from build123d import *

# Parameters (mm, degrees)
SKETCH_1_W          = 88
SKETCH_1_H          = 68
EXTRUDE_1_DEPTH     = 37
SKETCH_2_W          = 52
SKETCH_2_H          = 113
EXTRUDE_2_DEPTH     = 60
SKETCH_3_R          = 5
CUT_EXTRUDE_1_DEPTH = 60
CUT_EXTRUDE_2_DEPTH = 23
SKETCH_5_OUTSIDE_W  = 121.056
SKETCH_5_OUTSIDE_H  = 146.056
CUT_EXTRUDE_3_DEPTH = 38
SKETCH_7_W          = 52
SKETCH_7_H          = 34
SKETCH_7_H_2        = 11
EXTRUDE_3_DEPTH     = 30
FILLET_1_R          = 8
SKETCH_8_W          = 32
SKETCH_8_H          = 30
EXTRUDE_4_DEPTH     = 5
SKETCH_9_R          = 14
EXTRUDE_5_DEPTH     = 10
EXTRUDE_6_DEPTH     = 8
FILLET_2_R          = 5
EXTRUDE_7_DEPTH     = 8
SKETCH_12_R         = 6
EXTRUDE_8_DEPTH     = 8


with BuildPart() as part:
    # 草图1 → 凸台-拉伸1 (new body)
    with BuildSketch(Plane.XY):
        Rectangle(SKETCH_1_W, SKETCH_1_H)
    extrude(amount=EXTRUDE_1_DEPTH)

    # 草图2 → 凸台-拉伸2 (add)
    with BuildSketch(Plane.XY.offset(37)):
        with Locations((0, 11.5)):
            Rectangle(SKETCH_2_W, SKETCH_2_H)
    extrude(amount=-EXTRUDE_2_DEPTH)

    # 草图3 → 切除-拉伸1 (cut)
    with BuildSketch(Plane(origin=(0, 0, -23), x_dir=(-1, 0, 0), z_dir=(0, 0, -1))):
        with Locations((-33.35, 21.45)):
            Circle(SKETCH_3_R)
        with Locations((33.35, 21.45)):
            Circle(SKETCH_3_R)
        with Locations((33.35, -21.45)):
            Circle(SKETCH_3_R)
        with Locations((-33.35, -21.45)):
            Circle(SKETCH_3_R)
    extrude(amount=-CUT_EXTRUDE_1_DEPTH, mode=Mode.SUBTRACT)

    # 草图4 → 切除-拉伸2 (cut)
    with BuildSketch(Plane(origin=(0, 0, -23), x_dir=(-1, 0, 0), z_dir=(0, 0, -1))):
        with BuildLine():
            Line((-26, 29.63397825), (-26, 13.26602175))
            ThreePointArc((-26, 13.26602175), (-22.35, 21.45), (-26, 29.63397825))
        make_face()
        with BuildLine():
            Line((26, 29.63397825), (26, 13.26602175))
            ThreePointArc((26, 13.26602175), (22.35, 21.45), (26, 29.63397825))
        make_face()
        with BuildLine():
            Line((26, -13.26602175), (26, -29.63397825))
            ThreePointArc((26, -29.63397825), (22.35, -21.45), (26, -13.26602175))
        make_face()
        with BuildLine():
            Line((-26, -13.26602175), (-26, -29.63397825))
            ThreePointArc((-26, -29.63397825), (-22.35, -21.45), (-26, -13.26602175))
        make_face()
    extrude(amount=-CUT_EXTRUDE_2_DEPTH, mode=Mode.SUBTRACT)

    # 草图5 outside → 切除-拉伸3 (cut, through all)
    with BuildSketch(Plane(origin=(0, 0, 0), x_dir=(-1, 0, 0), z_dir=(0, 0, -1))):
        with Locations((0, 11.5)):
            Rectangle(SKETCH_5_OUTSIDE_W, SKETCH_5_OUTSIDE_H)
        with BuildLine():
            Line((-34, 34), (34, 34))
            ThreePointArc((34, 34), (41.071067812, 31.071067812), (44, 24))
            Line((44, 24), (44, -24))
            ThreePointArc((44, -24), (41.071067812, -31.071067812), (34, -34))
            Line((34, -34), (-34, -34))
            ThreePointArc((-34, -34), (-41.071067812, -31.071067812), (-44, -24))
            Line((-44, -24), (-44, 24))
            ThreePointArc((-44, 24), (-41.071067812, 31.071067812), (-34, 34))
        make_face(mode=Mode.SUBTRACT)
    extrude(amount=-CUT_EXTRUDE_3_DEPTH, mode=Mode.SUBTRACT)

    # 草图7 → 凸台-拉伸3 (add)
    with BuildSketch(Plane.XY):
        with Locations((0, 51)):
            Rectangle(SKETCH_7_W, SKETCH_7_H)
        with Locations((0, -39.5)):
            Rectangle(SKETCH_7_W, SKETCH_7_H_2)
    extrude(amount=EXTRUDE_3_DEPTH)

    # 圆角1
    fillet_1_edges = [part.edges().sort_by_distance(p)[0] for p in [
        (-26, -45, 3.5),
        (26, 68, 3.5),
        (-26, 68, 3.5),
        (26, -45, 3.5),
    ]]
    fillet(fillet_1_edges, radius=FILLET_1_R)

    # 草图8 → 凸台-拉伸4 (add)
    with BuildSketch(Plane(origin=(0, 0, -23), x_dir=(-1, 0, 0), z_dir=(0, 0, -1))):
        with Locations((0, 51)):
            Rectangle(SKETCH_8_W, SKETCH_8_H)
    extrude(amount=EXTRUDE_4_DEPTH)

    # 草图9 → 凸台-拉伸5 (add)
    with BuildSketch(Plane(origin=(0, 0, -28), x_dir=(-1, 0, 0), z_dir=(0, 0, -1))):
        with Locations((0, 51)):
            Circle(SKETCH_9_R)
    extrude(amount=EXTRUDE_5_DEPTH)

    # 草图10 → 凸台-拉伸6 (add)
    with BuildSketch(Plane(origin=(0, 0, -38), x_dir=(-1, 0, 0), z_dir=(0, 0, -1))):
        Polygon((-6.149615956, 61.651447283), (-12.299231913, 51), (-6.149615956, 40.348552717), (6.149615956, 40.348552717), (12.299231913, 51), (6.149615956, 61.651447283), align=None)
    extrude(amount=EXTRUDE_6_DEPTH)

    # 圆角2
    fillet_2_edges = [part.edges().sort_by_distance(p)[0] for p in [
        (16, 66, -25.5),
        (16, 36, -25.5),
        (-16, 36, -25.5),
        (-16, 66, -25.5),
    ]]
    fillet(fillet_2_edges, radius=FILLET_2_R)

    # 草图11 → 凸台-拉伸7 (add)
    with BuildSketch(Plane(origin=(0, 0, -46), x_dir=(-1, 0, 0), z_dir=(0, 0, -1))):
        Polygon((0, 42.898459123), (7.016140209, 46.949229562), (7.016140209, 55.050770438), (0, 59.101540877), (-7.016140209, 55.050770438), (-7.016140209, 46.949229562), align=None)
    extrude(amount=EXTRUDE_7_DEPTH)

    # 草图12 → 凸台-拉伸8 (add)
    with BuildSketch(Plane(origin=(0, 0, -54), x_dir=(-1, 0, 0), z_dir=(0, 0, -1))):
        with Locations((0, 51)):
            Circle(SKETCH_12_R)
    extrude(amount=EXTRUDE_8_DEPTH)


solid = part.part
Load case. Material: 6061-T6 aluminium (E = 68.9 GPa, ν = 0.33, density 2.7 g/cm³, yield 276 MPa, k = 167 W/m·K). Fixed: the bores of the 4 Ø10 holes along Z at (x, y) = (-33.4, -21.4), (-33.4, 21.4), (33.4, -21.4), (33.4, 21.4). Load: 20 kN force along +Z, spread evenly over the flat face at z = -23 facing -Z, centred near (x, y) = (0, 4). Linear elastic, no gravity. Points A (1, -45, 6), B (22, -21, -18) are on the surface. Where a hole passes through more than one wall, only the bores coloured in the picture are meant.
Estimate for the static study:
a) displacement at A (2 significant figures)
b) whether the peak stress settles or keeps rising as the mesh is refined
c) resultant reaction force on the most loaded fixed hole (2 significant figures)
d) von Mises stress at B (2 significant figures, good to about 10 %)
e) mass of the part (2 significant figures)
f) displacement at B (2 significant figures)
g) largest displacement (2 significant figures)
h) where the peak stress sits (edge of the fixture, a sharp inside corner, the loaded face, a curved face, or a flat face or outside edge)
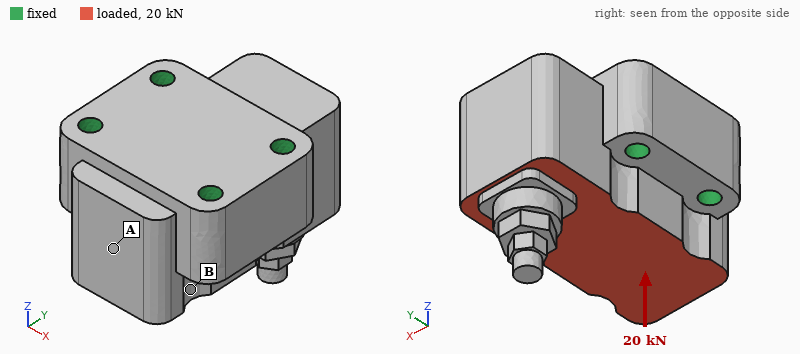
3.7 µm
keeps rising
5.8 kN
5.5 MPa
1.1 kg
4.0 µm
9.8 µm
edge of the fixture
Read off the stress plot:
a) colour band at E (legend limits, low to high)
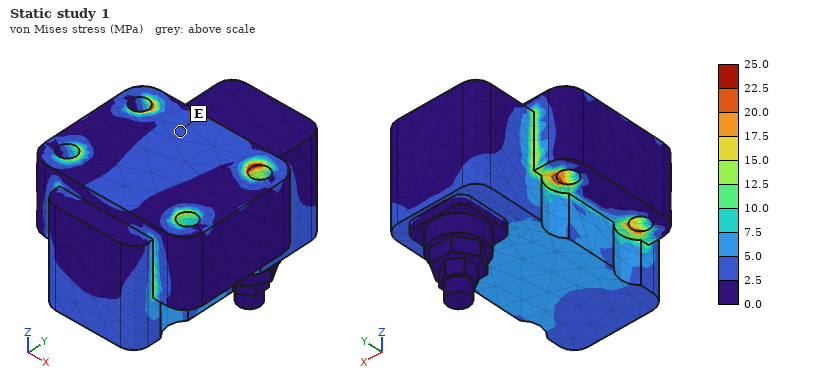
2.5 to 5.0 MPa
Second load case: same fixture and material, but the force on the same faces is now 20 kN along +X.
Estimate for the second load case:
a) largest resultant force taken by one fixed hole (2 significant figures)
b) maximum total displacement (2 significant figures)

7.9 kN
20 µm
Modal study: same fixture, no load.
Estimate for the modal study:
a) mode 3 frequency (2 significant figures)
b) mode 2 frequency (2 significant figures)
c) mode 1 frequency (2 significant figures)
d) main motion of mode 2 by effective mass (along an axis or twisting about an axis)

13 kHz
8700 Hz
6200 Hz
along X
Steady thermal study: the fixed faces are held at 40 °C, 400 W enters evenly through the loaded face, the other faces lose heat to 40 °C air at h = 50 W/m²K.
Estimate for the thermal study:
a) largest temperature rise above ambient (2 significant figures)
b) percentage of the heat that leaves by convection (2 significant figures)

23 K
3.8 %
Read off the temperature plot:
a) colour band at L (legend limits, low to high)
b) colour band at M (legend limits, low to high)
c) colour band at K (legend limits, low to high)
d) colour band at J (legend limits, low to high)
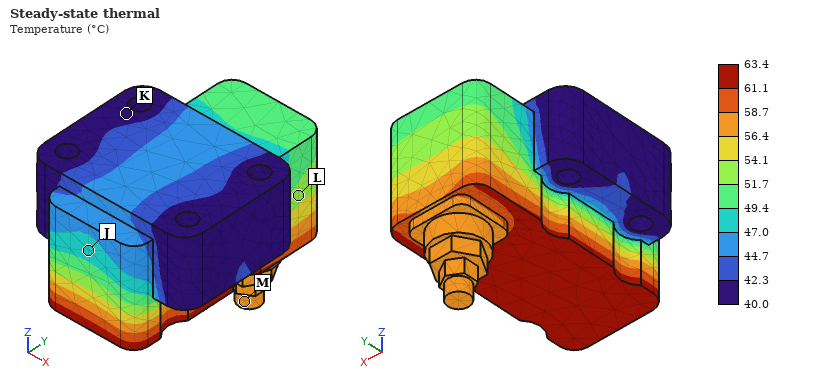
51.7 to 54.1 °C
56.4 to 58.7 °C
40.0 to 42.3 °C
47.0 to 49.4 °C
